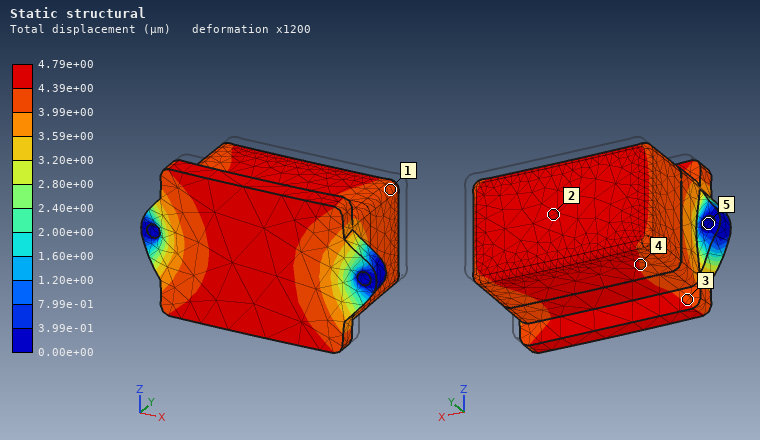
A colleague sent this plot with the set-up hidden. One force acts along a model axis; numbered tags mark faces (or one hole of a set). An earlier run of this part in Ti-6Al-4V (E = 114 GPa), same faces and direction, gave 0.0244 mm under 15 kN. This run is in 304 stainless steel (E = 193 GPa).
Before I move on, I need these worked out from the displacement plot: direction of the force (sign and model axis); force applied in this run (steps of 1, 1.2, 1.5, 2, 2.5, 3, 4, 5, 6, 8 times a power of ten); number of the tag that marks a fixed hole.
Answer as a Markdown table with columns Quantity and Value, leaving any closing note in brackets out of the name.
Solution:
| Quantity | Value |
|---|---|
| direction of the force | -Y |
| force applied in this run | 5 kN |
| number of the tag that marks a fixed hole | 5 |
